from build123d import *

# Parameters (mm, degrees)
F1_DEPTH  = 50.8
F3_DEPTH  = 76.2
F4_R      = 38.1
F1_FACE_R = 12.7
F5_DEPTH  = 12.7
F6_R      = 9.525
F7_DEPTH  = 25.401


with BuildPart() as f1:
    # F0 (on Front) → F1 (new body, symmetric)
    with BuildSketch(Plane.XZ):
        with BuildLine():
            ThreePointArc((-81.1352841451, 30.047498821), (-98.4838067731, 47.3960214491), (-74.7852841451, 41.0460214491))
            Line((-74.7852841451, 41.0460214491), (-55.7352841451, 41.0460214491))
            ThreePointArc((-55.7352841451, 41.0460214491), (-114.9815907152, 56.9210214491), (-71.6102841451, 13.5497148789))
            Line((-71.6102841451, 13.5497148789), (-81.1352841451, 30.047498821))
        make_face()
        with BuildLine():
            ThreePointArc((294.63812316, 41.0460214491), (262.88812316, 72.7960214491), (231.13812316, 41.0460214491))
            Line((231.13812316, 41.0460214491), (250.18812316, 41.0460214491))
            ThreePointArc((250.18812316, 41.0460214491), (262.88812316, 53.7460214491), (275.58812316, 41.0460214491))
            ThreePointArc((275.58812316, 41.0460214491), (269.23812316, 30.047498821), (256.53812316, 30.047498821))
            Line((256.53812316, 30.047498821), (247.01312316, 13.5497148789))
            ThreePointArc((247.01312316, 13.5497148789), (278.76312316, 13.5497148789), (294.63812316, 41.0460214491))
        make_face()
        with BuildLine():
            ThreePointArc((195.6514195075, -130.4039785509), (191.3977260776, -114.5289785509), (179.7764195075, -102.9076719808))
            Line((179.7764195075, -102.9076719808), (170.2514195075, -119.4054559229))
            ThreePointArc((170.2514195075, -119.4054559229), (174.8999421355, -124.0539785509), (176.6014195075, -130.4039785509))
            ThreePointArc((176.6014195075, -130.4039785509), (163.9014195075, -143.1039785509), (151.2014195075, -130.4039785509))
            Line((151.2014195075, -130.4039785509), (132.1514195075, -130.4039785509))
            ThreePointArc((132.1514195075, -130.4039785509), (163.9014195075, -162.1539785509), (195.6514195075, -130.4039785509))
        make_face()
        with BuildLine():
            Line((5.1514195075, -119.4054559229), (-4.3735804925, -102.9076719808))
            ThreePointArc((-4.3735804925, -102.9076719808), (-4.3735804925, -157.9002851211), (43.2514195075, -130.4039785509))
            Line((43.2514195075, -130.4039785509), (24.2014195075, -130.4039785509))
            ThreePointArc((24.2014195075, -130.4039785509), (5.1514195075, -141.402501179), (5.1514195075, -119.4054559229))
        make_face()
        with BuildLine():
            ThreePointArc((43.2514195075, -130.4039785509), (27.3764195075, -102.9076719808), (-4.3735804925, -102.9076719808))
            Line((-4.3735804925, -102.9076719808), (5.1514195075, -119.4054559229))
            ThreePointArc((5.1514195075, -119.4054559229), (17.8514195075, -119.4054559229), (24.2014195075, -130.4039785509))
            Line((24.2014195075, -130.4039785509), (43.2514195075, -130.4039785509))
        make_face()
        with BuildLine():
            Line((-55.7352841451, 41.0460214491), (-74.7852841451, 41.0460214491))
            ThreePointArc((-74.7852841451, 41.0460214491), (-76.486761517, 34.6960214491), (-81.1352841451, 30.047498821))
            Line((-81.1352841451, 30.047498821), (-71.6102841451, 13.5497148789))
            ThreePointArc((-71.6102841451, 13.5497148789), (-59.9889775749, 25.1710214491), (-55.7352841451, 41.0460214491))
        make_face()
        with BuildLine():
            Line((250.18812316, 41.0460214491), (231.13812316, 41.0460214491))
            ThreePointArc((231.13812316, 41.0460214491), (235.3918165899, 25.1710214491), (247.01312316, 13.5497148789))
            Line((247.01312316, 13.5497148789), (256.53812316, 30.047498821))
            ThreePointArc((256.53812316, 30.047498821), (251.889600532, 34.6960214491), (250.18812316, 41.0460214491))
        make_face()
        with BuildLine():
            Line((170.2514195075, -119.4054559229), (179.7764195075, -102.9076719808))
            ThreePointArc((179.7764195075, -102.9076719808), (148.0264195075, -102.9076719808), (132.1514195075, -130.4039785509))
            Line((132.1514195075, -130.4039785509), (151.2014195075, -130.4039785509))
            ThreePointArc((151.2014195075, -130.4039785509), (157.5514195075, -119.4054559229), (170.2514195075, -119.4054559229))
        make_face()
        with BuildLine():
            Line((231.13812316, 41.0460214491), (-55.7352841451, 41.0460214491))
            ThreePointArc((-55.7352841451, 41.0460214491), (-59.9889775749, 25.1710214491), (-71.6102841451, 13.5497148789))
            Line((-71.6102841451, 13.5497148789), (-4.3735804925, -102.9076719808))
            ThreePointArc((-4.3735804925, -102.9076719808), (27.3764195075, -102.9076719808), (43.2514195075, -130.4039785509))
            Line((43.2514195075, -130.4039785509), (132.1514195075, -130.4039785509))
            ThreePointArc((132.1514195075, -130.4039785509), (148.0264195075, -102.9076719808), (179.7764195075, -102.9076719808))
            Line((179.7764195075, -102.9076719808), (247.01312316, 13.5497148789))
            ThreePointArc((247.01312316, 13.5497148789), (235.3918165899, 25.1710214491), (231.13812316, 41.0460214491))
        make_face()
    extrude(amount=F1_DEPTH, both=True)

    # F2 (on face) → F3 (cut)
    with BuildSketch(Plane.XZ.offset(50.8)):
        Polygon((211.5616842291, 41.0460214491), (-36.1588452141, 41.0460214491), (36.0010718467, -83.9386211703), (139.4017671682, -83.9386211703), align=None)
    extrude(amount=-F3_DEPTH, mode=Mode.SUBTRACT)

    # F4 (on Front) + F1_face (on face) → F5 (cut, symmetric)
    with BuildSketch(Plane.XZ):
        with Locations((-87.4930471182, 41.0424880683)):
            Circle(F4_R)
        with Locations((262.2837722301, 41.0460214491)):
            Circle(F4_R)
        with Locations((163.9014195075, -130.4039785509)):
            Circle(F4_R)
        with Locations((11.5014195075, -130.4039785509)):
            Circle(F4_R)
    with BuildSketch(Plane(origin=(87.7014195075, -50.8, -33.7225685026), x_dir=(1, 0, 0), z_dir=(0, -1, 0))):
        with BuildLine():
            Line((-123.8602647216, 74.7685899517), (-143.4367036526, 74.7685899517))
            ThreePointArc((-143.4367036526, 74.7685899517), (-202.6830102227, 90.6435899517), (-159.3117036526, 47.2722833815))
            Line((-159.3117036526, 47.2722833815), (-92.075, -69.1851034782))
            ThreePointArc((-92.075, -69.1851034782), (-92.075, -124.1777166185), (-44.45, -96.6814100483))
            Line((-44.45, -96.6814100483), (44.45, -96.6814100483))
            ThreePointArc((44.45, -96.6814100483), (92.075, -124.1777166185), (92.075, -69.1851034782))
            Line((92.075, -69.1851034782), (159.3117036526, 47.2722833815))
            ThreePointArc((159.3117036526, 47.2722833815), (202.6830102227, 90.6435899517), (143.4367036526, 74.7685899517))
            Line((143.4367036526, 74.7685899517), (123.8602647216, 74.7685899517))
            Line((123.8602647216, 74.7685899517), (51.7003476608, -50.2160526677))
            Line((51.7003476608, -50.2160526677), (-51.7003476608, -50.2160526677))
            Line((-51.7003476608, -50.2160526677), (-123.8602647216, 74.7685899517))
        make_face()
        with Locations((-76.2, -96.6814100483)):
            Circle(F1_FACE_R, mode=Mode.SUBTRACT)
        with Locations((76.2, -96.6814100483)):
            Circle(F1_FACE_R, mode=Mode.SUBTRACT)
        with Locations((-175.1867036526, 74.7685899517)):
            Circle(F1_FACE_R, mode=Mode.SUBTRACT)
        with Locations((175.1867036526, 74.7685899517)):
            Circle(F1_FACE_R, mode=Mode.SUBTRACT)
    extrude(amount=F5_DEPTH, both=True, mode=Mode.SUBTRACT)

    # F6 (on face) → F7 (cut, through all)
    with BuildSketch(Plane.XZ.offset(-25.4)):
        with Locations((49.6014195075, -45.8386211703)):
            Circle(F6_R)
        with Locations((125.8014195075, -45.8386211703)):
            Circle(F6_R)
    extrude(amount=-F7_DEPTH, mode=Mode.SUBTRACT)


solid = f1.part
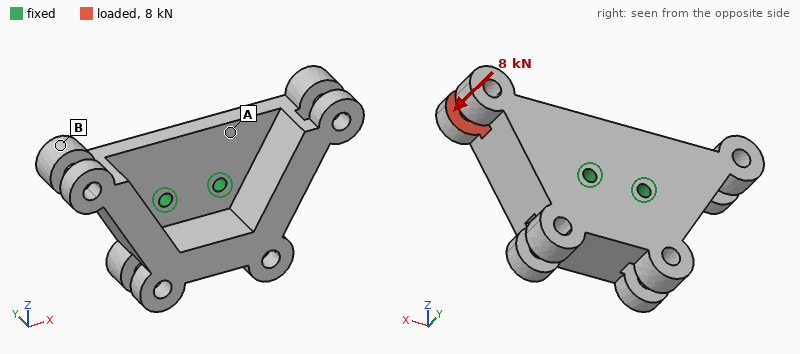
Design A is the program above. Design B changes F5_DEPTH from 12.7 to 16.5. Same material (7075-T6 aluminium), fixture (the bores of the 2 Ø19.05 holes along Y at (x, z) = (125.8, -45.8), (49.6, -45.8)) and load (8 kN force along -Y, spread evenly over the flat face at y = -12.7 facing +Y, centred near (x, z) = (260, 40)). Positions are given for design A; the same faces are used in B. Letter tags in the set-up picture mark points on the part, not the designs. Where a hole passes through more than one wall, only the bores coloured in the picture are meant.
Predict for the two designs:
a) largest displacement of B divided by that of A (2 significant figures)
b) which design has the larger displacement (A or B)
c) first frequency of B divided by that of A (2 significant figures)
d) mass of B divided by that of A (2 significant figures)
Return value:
1.5
B
1.1
0.93
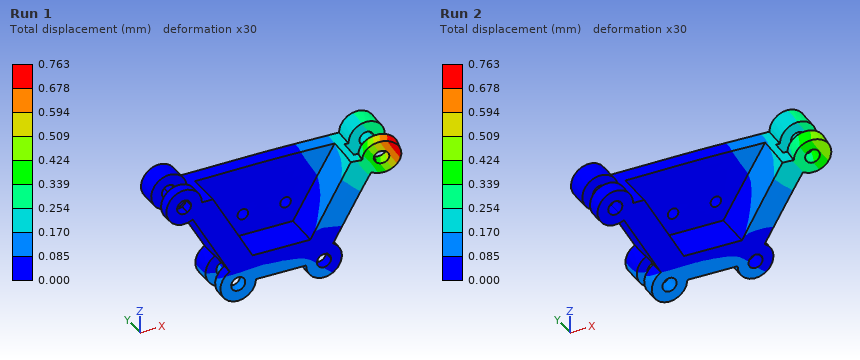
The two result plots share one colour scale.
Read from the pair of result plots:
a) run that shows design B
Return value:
Run 1
